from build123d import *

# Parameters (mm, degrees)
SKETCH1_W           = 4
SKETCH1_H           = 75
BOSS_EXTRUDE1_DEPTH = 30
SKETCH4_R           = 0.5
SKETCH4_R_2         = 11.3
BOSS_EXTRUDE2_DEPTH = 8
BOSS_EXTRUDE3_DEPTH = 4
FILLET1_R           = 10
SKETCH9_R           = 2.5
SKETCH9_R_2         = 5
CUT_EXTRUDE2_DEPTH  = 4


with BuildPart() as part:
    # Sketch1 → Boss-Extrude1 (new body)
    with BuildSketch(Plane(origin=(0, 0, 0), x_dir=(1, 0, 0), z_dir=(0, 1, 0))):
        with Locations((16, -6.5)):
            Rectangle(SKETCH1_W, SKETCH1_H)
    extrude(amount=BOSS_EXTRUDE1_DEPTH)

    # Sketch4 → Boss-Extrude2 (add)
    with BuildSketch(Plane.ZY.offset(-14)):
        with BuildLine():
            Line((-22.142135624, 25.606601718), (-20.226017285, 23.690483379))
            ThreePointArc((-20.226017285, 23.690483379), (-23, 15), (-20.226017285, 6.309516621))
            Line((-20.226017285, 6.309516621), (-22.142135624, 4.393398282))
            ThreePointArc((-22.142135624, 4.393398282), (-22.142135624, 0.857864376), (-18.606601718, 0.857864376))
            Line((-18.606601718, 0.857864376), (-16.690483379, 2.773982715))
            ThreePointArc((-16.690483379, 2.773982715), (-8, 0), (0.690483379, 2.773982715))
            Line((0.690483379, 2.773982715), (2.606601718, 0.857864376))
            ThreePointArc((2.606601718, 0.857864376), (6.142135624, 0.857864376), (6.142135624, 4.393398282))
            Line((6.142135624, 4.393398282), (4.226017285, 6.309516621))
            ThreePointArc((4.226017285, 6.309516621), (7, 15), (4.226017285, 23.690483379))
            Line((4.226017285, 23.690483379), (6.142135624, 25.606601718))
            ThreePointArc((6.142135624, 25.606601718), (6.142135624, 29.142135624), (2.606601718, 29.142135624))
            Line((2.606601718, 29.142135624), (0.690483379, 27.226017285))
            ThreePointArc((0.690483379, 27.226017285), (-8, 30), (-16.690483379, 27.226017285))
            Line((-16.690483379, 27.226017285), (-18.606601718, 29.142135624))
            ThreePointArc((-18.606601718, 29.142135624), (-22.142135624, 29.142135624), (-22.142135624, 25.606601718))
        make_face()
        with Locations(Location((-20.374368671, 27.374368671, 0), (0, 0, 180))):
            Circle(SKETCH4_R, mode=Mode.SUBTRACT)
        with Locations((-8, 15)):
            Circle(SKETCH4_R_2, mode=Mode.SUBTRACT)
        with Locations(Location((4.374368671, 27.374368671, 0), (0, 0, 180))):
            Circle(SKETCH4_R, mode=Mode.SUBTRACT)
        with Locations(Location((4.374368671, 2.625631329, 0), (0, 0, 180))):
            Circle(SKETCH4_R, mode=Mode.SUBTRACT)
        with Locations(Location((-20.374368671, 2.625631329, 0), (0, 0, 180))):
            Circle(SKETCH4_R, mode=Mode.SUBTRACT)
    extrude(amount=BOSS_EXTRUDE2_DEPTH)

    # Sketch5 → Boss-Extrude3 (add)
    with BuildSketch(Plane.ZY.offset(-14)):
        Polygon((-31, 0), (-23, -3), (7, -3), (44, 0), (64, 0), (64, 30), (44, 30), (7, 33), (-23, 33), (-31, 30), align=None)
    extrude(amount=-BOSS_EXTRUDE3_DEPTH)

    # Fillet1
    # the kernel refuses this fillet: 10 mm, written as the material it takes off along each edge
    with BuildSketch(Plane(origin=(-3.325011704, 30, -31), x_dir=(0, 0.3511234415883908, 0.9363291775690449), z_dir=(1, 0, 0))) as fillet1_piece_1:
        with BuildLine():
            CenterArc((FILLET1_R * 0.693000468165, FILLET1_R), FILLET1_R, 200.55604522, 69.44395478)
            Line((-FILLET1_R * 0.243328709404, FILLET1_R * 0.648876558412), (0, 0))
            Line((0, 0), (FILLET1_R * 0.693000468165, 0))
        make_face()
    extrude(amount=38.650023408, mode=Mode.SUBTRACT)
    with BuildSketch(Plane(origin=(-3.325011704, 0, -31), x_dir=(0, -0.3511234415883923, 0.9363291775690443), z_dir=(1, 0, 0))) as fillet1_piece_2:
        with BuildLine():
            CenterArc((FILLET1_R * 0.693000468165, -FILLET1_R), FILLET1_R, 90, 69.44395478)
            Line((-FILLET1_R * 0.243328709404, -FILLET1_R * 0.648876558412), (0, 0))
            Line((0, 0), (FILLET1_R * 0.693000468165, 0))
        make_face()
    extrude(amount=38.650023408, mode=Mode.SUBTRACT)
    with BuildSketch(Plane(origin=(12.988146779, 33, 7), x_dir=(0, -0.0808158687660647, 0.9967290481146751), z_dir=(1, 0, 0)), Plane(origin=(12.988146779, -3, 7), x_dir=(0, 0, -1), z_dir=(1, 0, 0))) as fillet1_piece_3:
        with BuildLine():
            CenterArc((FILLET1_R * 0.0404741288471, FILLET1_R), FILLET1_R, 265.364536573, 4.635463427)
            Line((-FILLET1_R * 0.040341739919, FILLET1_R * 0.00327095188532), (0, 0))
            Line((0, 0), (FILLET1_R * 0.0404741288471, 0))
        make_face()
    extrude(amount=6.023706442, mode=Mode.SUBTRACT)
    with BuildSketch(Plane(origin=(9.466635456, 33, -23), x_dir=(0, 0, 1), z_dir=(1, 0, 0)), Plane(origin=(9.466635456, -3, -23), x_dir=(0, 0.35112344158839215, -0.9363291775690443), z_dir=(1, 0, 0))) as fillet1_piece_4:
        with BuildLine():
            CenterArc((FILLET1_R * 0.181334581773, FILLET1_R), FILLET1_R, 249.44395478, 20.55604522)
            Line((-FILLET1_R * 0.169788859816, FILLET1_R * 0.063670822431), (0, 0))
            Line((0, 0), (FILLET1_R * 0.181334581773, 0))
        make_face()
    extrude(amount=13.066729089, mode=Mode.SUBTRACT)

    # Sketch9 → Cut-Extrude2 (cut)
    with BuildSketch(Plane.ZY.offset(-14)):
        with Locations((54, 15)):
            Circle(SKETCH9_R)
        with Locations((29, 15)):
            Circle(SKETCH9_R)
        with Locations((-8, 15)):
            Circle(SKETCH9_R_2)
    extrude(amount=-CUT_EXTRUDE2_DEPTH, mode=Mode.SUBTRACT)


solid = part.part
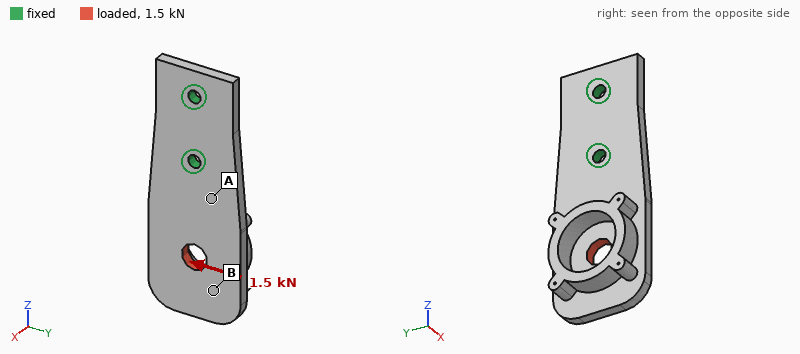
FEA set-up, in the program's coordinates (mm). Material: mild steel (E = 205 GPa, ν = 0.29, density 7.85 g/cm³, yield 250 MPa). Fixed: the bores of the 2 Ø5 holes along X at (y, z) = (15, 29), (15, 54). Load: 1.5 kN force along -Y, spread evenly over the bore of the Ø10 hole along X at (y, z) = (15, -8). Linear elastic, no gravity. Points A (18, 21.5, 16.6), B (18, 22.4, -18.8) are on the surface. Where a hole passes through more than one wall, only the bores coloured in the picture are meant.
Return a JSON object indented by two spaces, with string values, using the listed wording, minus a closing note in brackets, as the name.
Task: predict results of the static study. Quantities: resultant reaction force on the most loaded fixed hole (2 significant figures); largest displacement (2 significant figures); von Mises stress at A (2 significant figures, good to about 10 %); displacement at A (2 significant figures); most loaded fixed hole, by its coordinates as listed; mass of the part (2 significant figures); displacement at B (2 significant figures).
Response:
{
  "resultant reaction force on the most loaded fixed hole": "3.2 kN",
  "largest displacement": "51 µm",
  "von Mises stress at A": "32 MPa",
  "displacement at A": "9.8 µm",
  "most loaded fixed hole, by its coordinates as listed": "(15, 29)",
  "mass of the part": "120 g",
  "displacement at B": "41 µm"
}
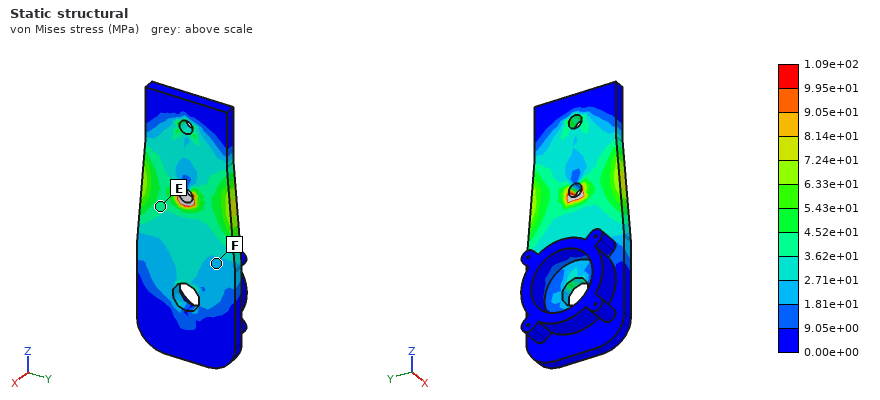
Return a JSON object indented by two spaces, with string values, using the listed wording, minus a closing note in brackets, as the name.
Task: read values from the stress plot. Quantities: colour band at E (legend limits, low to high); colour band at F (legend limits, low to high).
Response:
{
  "colour band at E": "3.62e+01 to 4.52e+01 MPa",
  "colour band at F": "1.81e+01 to 2.71e+01 MPa"
}
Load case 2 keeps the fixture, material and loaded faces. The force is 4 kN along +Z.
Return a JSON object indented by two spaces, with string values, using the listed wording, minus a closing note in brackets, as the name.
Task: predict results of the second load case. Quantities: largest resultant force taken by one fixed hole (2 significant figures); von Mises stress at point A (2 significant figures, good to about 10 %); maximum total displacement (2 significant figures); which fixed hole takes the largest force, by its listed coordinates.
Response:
{
  "largest resultant force taken by one fixed hole": "3.2 kN",
  "von Mises stress at point A": "34 MPa",
  "maximum total displacement": "11 µm",
  "which fixed hole takes the largest force, by its listed coordinates": "(15, 29)"
}
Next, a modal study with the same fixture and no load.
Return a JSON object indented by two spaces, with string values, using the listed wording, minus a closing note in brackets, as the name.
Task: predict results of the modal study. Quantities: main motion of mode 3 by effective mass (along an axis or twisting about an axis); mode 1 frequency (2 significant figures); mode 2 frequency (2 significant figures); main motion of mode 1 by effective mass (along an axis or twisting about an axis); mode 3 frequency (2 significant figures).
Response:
{
  "main motion of mode 3 by effective mass": "along Y",
  "mode 1 frequency": "800 Hz",
  "mode 2 frequency": "2600 Hz",
  "main motion of mode 1 by effective mass": "along X",
  "mode 3 frequency": "3800 Hz"
}
